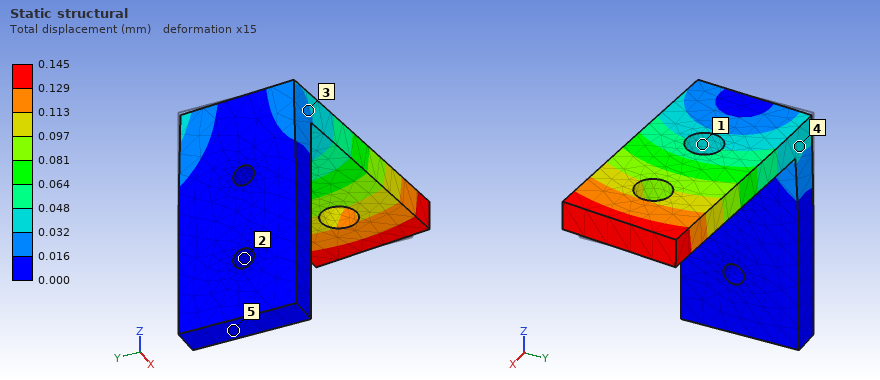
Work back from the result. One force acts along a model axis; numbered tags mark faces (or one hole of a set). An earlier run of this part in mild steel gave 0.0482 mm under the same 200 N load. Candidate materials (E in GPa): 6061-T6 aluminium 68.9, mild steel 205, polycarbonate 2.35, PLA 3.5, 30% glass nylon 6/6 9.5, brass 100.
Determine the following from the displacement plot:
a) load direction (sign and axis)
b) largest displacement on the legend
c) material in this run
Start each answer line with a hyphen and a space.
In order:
- -Y
- 0.145 mm
- 6061-T6 aluminium
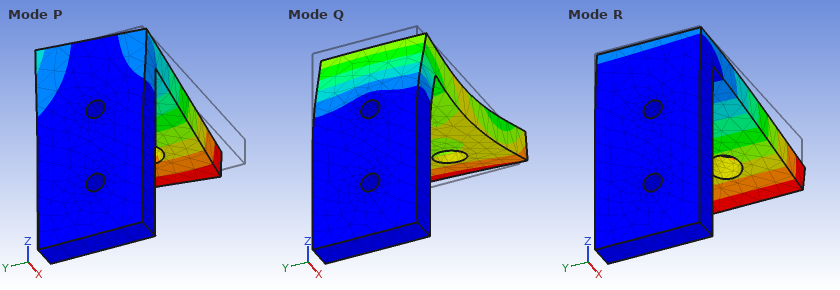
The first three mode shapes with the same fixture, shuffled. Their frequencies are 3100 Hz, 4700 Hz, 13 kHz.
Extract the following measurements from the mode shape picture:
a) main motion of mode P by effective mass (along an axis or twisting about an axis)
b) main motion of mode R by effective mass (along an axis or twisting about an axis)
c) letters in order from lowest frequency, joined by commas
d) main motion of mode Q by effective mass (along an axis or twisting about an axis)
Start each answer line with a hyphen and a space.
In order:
- along Y
- along Z
- R, P, Q
- along X
